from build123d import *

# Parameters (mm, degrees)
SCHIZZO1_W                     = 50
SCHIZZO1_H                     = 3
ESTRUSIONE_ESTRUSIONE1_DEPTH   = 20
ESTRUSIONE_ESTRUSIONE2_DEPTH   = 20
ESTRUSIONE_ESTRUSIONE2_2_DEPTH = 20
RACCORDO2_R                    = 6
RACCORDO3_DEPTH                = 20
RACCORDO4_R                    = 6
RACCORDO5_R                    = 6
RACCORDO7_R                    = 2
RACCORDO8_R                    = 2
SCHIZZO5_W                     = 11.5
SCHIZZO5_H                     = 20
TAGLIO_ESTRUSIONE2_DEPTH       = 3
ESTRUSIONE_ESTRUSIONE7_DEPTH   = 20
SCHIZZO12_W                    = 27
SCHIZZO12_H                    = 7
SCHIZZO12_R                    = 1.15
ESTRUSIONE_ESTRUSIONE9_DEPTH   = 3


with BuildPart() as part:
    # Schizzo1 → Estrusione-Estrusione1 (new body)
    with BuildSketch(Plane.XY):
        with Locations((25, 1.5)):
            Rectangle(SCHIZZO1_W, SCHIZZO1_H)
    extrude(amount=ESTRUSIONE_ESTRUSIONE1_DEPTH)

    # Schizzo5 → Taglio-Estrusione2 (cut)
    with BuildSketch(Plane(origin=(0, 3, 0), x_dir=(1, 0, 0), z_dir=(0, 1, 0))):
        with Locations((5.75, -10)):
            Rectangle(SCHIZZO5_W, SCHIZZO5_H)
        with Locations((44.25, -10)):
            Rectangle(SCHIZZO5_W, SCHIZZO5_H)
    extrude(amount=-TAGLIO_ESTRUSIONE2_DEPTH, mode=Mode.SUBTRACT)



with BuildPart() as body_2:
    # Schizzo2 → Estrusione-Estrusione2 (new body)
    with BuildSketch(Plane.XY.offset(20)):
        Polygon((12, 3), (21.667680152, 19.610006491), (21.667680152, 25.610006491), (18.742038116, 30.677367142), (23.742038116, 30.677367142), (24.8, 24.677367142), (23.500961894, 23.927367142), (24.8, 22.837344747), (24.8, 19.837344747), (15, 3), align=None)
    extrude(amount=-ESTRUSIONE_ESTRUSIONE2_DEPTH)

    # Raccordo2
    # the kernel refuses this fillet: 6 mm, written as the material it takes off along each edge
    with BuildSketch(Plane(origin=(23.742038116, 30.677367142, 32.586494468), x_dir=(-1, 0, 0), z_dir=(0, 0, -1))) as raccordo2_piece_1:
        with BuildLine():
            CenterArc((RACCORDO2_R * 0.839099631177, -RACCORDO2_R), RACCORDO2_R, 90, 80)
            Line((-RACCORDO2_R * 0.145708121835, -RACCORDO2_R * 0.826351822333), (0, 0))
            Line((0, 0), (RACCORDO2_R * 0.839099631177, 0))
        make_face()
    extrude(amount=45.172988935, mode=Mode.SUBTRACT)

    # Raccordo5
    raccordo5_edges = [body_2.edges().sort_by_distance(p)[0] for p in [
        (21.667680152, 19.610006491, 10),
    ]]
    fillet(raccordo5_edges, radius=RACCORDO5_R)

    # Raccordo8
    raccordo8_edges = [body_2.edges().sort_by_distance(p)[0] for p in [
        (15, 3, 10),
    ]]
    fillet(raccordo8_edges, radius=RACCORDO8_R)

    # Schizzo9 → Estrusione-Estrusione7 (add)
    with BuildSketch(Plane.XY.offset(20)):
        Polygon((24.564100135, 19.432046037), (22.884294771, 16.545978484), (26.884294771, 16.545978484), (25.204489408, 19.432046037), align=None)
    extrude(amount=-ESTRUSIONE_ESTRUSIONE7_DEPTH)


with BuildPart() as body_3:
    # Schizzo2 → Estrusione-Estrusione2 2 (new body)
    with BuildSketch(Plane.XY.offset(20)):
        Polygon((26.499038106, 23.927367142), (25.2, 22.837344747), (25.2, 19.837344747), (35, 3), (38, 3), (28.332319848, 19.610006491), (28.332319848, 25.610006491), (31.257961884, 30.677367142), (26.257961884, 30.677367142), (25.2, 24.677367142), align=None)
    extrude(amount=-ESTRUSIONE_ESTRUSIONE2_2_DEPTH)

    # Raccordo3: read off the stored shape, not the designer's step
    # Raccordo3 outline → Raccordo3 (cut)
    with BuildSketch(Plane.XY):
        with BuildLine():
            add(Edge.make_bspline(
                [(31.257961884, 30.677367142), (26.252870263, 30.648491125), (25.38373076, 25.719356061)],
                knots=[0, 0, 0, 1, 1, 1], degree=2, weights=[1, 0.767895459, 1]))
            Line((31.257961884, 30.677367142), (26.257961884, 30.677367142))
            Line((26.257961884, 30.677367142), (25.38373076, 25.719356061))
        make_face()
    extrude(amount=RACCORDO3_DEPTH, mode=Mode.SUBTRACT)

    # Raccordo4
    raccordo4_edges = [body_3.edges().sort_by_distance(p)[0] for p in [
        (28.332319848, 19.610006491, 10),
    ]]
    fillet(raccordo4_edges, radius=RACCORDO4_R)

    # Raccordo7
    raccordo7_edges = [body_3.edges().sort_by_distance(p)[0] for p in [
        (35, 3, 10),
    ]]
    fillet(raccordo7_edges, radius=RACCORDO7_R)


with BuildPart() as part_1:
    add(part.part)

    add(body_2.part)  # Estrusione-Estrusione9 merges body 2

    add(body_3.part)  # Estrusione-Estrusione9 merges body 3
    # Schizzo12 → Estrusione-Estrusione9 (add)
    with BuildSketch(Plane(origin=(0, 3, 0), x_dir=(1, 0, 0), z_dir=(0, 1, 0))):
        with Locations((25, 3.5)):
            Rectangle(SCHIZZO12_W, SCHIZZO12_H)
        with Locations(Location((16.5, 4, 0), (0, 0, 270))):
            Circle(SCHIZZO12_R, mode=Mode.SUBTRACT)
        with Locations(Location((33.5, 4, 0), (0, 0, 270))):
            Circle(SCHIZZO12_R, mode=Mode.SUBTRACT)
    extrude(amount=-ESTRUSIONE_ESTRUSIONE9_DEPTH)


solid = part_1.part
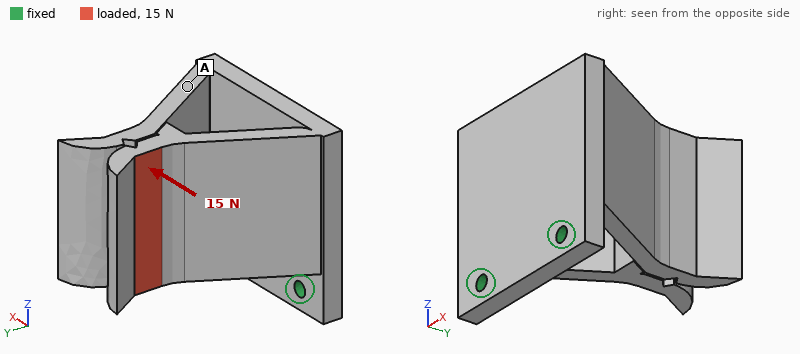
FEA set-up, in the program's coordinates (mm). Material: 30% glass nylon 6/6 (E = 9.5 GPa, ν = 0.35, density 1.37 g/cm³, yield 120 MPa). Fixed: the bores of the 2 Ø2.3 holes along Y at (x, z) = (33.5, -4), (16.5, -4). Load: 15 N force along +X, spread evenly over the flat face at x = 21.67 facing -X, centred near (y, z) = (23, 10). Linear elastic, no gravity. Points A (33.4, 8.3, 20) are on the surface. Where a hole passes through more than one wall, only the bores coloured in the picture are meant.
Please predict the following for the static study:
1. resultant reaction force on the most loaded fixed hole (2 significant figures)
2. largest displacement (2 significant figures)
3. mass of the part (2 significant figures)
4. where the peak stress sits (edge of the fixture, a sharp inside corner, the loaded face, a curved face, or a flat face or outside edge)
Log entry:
19 N
0.58 mm
7.7 g
a flat face or outside edge
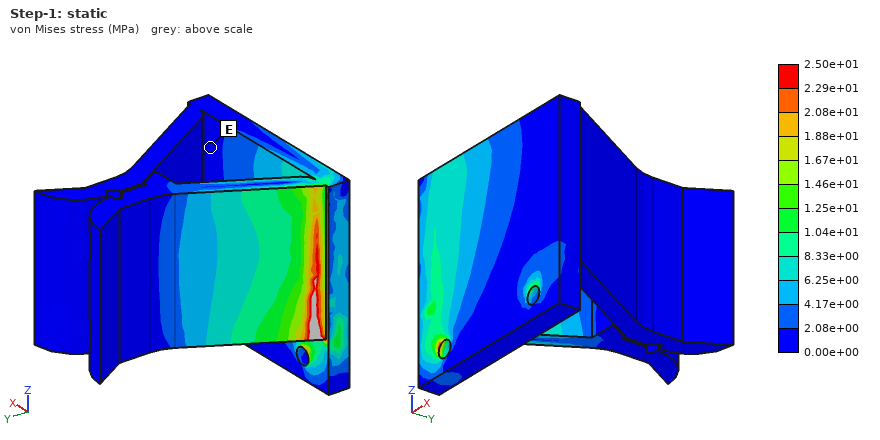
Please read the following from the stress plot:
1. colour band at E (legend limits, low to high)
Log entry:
0.00e+00 to 2.08e+00 MPa
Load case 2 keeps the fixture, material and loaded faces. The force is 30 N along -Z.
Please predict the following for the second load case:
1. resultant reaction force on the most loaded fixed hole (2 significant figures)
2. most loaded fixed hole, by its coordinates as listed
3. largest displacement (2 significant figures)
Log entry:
20 N
(16.5, -4)
0.55 mm
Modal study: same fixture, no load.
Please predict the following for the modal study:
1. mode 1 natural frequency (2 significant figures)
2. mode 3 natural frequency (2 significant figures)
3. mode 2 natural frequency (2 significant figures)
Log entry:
740 Hz
870 Hz
770 Hz
